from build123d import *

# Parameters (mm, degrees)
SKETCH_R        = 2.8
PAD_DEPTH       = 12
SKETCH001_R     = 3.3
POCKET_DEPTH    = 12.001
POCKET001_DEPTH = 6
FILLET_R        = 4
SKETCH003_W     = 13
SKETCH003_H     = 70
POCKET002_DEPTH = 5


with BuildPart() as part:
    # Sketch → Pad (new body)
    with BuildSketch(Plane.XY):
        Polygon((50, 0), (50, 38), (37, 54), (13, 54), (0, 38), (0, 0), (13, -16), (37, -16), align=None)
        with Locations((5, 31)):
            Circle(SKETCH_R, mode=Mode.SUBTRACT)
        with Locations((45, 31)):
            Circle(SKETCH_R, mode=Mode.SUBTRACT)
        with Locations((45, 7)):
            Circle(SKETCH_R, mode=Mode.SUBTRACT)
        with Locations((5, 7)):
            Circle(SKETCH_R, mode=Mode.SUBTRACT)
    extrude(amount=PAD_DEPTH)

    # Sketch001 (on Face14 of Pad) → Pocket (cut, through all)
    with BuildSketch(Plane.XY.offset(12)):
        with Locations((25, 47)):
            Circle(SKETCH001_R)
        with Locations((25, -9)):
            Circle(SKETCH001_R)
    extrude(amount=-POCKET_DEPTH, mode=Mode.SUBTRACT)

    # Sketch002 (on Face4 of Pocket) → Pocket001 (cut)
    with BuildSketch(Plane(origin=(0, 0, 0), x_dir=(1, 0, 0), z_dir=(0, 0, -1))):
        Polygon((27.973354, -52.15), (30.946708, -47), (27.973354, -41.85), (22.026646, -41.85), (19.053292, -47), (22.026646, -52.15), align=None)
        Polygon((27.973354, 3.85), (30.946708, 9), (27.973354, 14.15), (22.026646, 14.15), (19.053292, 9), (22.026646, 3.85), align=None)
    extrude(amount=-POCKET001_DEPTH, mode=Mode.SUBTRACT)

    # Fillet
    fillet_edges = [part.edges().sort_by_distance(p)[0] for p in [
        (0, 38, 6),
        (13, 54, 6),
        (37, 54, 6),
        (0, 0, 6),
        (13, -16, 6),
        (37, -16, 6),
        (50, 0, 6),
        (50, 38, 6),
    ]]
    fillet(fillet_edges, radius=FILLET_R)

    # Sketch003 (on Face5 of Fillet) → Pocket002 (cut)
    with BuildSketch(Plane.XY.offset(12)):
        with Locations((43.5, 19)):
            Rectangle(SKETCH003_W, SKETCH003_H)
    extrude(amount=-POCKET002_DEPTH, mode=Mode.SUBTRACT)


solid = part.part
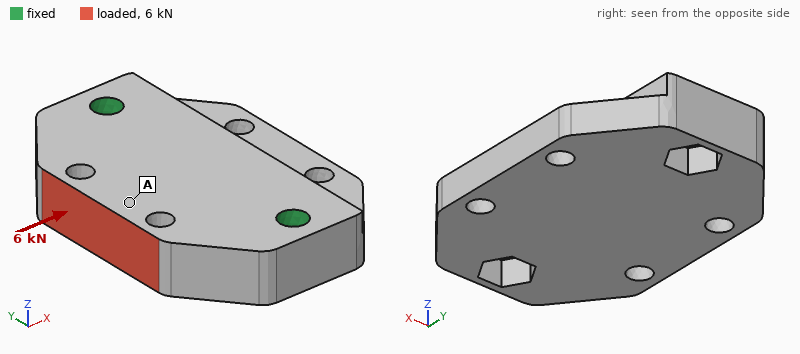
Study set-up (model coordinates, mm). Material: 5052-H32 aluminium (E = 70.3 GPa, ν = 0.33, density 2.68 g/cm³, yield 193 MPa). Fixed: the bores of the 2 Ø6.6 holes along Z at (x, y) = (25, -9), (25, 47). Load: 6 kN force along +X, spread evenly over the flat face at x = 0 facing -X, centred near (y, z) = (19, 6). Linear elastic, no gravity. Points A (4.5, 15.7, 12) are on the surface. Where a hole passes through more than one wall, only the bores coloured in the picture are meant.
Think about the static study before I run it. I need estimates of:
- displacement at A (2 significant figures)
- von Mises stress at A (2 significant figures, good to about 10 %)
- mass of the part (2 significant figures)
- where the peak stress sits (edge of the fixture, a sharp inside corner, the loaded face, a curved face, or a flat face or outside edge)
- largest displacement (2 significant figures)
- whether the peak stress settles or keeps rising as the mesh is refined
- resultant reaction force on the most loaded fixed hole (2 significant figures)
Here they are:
17 µm
14 MPa
83 g
edge of the fixture
27 µm
keeps rising
3.1 kN
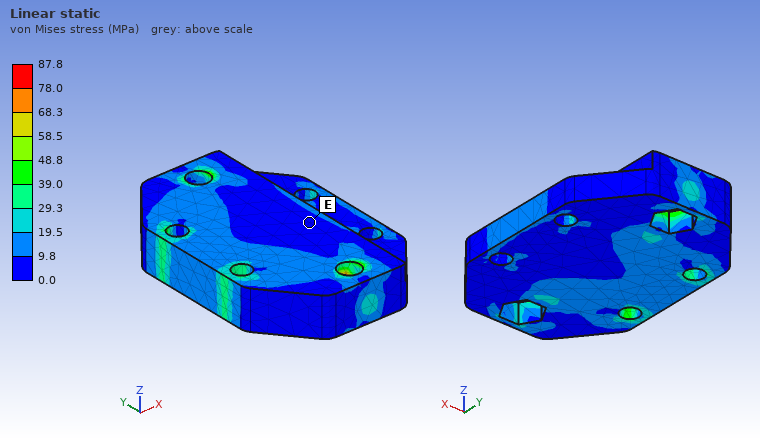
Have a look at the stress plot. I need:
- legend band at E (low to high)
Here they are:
0.0 to 9.8 MPa
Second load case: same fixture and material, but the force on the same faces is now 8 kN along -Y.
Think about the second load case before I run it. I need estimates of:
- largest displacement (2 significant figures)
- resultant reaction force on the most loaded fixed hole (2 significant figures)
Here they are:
23 µm
5.3 kN
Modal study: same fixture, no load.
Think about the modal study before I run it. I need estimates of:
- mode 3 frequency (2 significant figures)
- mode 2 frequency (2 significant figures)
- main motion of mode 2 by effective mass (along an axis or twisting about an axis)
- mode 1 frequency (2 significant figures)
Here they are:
16 kHz
9600 Hz
along Z
6200 Hz
